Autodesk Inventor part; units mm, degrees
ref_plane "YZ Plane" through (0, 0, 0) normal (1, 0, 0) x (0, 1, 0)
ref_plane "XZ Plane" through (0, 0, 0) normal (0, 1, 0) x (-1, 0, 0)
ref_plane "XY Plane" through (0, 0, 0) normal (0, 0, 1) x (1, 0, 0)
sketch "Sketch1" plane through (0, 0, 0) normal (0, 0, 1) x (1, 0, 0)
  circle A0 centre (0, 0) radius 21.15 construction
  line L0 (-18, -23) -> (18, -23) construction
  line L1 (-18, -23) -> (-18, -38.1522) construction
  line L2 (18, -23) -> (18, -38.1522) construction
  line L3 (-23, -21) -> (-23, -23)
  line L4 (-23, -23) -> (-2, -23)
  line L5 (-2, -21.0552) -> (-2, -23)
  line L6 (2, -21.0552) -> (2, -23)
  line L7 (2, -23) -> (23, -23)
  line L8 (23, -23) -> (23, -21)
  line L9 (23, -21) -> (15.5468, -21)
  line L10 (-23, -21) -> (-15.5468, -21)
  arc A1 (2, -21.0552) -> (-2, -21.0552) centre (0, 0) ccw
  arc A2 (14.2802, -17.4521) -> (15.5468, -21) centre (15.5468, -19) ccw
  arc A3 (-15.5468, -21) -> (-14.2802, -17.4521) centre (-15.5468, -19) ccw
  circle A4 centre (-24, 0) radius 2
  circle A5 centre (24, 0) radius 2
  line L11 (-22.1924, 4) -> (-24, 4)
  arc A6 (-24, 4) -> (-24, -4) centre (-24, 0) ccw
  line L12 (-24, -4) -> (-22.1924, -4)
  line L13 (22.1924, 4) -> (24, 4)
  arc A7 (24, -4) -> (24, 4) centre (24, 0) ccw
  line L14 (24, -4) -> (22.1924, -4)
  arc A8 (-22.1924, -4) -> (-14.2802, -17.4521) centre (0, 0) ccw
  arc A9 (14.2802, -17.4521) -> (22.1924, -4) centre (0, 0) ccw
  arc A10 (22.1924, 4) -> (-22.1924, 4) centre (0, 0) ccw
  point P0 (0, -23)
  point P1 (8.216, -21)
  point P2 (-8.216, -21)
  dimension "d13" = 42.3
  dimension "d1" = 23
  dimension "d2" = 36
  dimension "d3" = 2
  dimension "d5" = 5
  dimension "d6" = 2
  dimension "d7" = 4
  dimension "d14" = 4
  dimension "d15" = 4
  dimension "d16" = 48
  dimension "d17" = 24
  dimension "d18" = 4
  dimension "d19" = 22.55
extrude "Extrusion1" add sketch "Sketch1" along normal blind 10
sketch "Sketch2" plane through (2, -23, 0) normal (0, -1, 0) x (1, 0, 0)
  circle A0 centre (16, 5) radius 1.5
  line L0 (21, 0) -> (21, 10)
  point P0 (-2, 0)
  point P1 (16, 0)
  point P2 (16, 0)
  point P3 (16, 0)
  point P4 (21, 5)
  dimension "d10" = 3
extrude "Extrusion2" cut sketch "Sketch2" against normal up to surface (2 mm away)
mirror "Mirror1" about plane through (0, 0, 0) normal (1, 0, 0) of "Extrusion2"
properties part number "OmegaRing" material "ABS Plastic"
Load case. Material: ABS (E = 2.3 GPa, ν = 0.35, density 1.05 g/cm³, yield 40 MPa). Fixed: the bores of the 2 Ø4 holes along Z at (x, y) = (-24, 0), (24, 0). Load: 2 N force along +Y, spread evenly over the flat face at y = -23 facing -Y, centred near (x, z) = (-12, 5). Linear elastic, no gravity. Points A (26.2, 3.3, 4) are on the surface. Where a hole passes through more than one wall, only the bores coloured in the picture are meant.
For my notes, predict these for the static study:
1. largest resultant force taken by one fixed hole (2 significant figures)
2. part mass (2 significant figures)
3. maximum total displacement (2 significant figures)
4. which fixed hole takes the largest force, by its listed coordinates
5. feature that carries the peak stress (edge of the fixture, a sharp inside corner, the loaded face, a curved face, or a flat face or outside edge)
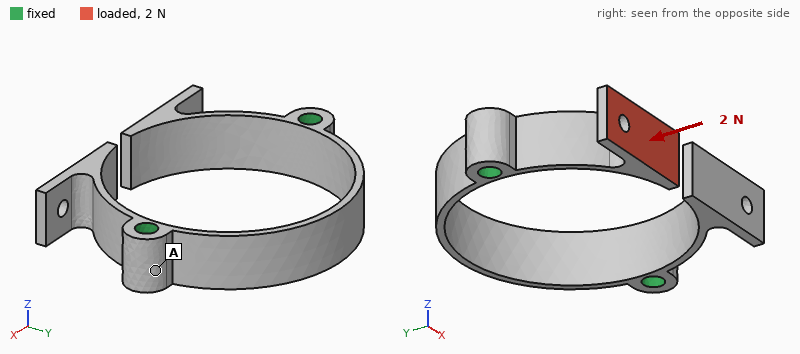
2.0 N
3.4 g
0.83 mm
(-24, 0)
a curved face
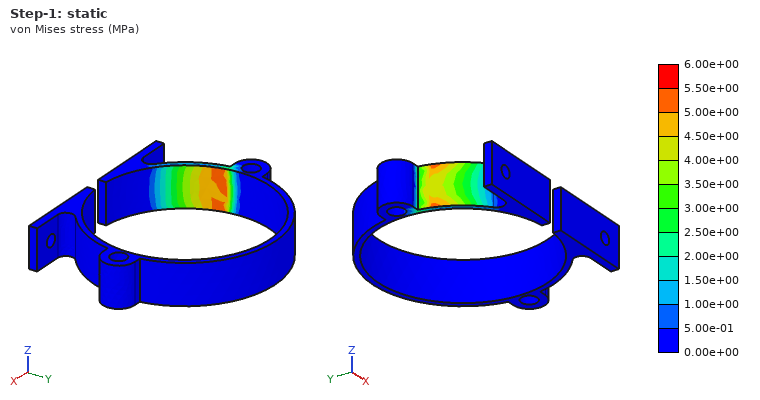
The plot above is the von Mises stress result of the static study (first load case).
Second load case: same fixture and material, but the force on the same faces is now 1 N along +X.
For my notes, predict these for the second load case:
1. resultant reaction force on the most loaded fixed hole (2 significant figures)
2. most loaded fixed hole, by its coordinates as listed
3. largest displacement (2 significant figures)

1.0 N
(-24, 0)
0.83 mm
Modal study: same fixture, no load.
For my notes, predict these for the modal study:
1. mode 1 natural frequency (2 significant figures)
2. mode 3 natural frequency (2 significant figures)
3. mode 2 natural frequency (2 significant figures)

250 Hz
810 Hz
250 Hz
